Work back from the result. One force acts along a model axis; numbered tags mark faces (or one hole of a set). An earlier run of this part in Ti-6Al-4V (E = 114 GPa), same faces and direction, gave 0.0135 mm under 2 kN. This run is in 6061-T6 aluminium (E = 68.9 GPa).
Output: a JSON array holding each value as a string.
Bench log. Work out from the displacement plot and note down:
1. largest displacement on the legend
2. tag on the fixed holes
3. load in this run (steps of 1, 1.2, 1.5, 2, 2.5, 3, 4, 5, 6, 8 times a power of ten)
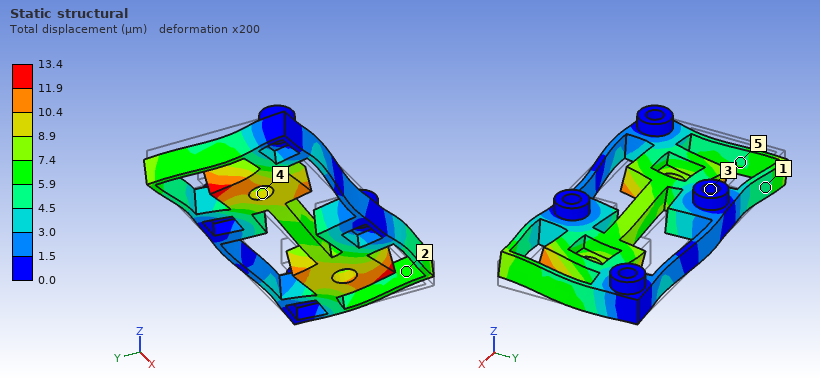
["13.4 µm", "3", "1.2 kN"]
